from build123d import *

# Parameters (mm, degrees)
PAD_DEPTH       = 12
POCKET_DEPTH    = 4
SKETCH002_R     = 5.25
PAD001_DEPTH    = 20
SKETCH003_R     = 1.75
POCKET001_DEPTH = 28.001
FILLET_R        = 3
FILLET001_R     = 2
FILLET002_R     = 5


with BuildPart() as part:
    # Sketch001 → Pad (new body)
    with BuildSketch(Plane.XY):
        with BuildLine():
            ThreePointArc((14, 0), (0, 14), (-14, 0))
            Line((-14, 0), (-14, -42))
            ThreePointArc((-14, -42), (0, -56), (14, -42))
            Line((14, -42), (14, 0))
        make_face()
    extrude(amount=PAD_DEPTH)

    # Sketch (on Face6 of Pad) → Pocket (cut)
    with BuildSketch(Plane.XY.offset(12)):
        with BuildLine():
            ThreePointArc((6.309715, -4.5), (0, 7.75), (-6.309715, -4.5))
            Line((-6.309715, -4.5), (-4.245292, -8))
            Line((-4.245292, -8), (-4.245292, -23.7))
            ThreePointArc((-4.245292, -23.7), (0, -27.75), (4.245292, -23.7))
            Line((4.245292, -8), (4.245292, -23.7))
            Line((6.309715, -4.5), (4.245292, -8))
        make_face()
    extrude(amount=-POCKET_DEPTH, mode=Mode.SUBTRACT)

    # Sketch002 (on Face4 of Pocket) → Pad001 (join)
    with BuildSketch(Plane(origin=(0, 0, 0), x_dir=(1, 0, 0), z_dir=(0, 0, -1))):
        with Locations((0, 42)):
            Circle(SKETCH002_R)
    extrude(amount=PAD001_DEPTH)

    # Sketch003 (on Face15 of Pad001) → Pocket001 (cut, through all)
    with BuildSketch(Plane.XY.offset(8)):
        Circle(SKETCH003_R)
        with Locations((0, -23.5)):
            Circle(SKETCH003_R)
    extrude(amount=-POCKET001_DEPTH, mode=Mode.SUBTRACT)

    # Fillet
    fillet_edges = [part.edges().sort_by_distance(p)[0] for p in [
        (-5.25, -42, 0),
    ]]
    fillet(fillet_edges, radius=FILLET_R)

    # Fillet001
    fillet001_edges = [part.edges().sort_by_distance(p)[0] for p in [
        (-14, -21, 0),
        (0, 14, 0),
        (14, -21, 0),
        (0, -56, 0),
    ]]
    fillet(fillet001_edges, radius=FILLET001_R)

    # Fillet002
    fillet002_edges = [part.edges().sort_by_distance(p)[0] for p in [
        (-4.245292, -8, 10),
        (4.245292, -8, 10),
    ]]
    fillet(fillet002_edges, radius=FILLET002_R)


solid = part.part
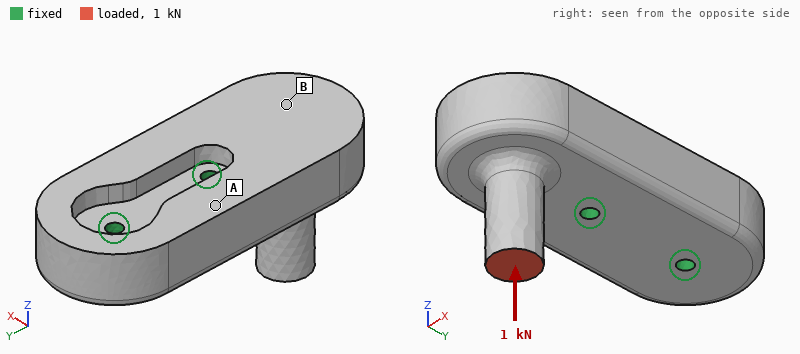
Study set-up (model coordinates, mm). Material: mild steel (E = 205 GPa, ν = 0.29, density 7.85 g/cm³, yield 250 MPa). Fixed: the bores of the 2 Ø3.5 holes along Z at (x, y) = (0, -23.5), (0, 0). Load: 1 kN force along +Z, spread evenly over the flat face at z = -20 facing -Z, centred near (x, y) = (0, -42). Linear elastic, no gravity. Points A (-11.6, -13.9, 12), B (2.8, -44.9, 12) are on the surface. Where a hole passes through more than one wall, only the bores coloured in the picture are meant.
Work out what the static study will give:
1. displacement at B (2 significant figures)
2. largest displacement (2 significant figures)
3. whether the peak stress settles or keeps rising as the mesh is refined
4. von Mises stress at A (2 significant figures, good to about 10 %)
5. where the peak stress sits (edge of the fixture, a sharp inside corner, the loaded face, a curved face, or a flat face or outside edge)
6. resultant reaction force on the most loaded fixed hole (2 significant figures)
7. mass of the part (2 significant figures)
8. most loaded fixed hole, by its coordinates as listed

8.6 µm
15 µm
keeps rising
13 MPa
edge of the fixture
1.5 kN
170 g
(0, -23.5)
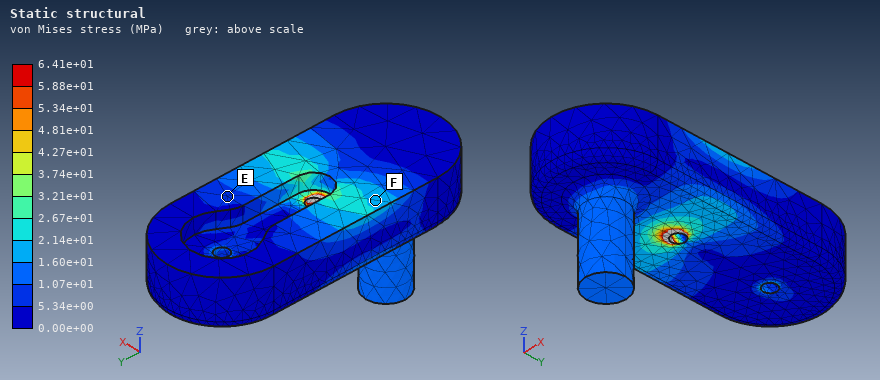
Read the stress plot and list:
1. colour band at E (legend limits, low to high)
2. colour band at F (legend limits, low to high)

5.34e+00 to 1.07e+01 MPa
1.60e+01 to 2.14e+01 MPa
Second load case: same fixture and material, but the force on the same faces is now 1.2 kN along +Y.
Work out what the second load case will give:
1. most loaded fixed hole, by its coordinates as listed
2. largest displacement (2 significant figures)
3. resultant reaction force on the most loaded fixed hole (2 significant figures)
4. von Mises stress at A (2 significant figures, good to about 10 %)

(0, -23.5)
63 µm
1.7 kN
20 MPa
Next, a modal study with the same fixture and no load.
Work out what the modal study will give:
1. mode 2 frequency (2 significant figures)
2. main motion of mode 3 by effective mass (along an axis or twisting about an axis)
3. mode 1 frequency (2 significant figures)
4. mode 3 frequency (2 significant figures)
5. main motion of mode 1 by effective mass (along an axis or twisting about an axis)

8300 Hz
along X
6000 Hz
10 kHz
along Z
